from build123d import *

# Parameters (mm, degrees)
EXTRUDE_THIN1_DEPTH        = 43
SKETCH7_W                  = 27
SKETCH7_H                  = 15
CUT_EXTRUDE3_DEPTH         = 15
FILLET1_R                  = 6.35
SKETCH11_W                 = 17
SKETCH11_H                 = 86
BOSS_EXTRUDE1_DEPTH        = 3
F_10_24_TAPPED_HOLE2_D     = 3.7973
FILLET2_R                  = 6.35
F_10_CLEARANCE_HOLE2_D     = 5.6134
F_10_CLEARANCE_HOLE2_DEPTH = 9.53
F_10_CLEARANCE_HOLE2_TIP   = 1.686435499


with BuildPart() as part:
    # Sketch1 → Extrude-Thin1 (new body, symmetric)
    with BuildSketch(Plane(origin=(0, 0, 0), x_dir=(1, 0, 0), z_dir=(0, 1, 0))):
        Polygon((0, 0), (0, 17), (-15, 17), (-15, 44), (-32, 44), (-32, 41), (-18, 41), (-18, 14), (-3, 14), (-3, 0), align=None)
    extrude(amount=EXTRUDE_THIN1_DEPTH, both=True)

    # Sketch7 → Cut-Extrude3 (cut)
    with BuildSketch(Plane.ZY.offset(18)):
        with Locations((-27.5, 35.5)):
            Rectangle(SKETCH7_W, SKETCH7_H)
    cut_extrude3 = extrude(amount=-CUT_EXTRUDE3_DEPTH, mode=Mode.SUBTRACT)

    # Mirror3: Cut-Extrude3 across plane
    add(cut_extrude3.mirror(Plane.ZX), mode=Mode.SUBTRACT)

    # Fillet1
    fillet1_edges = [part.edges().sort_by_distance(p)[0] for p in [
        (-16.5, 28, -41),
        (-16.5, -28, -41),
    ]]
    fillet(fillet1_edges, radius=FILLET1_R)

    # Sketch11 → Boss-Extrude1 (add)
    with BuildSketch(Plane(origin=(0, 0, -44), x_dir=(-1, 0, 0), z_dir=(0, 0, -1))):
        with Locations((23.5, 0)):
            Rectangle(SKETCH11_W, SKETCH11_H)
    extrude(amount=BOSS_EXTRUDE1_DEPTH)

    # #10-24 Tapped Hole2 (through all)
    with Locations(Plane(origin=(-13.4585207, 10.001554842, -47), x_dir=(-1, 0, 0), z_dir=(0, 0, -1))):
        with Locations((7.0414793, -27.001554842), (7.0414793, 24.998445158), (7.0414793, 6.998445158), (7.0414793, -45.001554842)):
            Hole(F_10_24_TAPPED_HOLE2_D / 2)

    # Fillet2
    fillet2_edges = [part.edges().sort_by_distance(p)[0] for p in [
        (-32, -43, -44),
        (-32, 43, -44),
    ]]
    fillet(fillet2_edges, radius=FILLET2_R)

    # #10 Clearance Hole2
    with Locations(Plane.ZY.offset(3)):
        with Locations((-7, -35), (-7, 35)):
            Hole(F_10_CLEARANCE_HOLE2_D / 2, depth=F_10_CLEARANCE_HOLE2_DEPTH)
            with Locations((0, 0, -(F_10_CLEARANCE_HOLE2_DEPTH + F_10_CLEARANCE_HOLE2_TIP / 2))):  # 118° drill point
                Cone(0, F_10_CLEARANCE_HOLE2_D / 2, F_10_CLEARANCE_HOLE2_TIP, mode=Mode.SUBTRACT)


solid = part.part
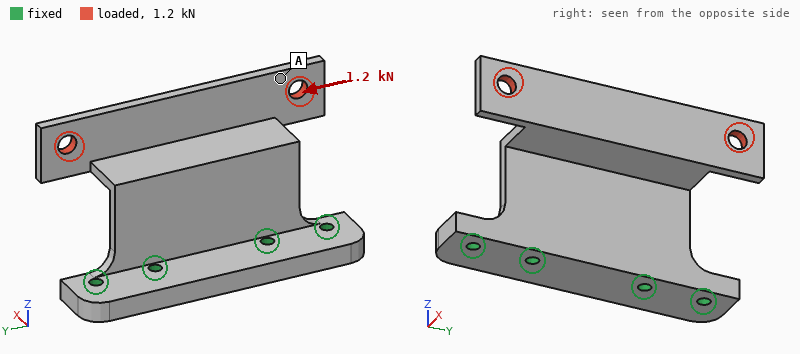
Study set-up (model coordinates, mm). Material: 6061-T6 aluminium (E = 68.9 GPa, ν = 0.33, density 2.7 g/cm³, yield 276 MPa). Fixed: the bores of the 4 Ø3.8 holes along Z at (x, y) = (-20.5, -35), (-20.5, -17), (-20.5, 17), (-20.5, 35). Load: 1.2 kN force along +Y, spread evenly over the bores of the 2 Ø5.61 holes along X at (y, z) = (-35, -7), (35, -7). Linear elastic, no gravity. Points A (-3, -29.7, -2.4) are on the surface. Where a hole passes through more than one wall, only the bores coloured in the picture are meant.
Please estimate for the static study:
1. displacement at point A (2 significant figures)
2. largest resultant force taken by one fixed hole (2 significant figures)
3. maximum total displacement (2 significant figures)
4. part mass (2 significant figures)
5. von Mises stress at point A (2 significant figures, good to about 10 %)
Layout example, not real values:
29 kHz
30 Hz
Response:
0.33 mm
860 N
0.50 mm
52 g
15 MPa
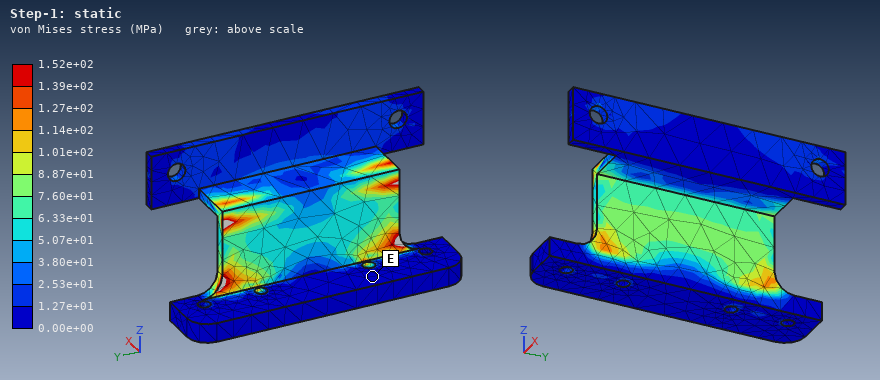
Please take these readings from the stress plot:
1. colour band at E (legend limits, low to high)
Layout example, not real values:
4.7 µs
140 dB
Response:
0.00e+00 to 1.27e+01 MPa
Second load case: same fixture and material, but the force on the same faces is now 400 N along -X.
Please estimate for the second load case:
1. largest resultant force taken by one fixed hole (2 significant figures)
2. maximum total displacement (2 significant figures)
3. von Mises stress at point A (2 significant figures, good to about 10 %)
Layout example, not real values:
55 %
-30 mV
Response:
260 N
1.2 mm
33 MPa
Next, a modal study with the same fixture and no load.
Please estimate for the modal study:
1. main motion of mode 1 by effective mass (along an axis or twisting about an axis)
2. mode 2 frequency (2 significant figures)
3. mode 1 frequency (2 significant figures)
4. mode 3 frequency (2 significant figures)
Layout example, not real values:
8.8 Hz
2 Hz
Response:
along X
1500 Hz
880 Hz
3100 Hz
